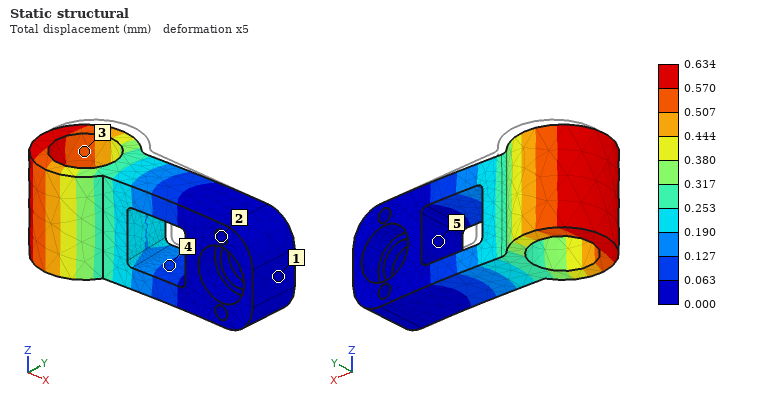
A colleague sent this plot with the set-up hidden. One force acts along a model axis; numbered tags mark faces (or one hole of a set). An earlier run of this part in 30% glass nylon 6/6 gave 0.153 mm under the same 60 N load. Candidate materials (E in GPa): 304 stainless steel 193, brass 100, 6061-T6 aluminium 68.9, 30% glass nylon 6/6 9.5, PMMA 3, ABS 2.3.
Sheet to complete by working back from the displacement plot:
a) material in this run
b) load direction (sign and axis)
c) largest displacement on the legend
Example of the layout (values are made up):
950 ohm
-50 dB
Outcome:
ABS
-Y
0.634 mm
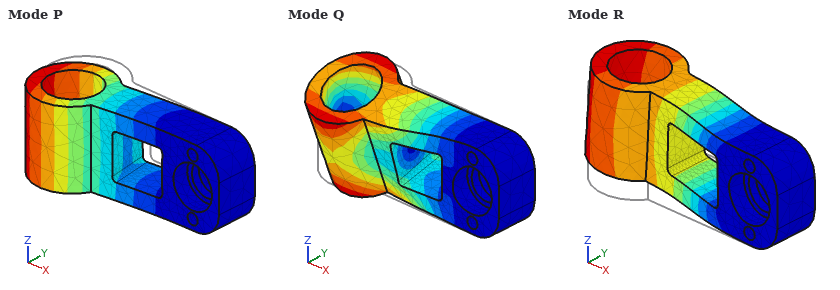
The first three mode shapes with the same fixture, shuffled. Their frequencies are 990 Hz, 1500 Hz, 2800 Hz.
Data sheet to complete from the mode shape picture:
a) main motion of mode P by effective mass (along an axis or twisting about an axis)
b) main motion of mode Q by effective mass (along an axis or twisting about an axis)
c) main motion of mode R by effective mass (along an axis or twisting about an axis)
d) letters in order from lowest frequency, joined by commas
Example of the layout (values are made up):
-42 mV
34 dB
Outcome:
along Y
twisting about X
along Z
P, R, Q
